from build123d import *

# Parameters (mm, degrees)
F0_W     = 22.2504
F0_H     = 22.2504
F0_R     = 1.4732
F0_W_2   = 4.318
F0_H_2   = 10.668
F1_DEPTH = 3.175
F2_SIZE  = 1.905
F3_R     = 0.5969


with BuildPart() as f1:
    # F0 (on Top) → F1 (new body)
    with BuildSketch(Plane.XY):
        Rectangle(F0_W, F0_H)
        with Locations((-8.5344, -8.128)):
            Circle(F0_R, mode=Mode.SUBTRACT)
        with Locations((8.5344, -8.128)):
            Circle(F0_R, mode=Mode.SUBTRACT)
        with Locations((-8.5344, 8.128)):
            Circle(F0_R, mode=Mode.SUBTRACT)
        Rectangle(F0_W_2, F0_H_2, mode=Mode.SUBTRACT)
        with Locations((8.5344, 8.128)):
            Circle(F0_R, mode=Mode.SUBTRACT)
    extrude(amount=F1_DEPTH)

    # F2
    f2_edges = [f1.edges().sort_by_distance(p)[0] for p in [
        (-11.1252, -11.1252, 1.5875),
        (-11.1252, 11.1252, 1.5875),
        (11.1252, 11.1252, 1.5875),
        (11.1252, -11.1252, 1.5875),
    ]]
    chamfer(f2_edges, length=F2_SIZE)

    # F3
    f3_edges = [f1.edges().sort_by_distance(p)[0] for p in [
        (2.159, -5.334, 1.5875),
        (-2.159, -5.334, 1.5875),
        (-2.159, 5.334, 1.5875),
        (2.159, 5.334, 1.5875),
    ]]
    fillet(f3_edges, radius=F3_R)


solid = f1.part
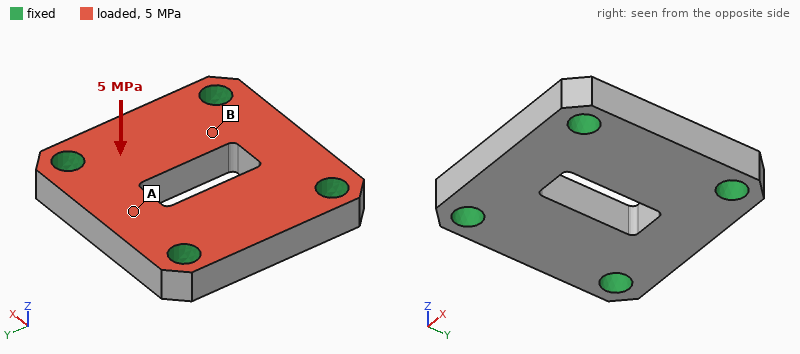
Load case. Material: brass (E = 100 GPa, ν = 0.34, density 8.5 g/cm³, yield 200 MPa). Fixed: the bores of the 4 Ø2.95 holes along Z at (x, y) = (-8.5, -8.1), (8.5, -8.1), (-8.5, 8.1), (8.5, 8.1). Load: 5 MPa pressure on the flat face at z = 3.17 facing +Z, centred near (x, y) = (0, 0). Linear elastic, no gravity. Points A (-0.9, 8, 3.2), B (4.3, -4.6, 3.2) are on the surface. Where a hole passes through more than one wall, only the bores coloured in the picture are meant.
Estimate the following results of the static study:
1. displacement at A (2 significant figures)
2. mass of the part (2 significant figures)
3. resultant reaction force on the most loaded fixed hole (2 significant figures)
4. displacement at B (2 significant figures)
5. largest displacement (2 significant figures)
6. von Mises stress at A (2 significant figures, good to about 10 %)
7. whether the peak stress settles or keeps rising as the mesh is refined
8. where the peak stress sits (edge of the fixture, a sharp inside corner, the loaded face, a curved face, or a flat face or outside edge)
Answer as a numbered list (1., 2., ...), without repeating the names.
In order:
1. 5.1 µm
2. 11 g
3. 520 N
4. 5.3 µm
5. 9.2 µm
6. 33 MPa
7. keeps rising
8. edge of the fixture
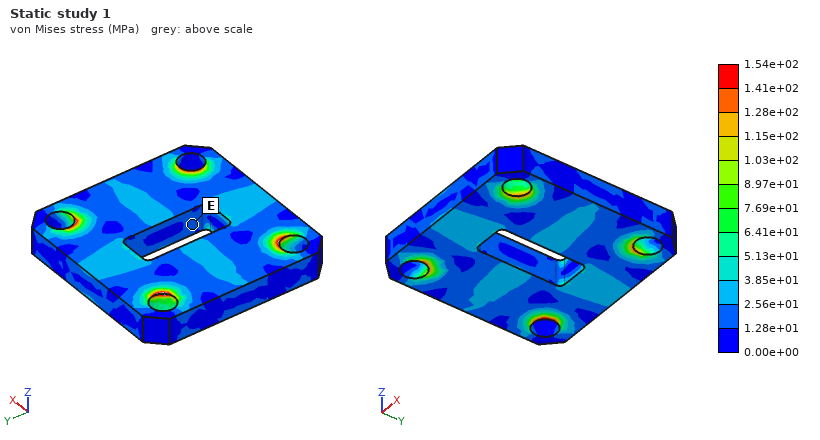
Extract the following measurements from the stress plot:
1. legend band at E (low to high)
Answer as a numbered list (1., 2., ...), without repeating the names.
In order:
1. 1.28e+01 to 2.56e+01 MPa
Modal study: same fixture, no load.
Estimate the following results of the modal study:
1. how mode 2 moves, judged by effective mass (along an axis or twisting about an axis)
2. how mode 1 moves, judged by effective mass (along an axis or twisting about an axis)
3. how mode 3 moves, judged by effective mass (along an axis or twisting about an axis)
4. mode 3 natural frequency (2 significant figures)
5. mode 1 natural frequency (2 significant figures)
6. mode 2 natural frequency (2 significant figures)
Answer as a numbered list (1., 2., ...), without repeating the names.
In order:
1. twisting about Y
2. along Z
3. twisting about X
4. 40 kHz
5. 30 kHz
6. 38 kHz
